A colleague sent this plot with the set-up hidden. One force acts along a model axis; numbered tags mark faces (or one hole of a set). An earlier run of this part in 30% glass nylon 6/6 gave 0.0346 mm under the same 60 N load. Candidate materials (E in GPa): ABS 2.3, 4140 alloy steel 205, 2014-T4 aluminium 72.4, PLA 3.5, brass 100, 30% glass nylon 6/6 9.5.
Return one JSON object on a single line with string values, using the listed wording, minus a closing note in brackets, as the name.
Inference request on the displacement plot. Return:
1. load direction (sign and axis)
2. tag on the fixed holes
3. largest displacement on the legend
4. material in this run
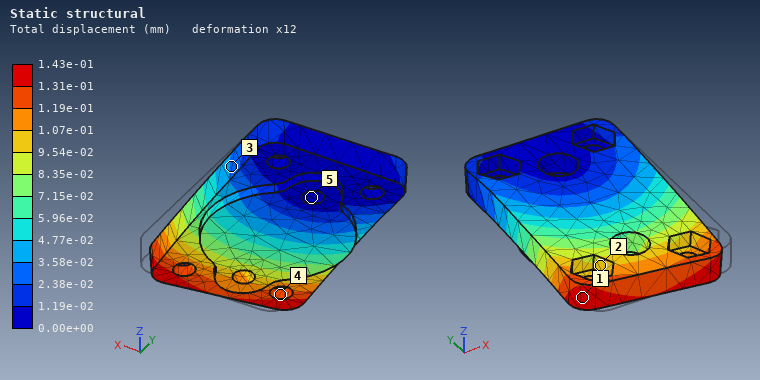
{"load direction": "-X", "tag on the fixed holes": "5", "largest displacement on the legend": "1.43e-01 mm", "material in this run": "ABS"}
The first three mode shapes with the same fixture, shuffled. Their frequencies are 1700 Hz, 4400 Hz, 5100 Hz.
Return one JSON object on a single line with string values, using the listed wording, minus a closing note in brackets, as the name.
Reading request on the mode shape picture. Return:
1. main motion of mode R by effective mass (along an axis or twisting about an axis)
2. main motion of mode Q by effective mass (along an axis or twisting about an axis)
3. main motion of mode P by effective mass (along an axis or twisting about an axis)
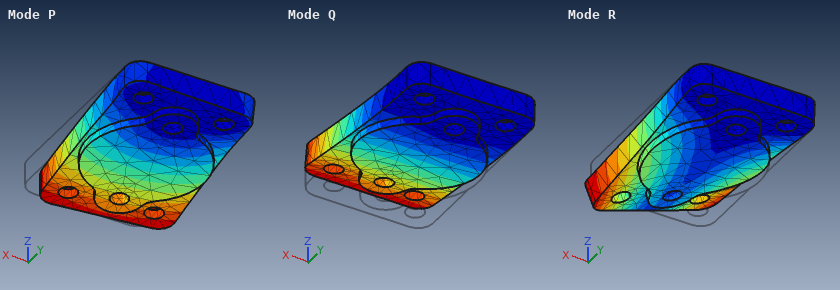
{"main motion of mode R by effective mass": "twisting about Y", "main motion of mode Q by effective mass": "along Z", "main motion of mode P by effective mass": "along X"}
